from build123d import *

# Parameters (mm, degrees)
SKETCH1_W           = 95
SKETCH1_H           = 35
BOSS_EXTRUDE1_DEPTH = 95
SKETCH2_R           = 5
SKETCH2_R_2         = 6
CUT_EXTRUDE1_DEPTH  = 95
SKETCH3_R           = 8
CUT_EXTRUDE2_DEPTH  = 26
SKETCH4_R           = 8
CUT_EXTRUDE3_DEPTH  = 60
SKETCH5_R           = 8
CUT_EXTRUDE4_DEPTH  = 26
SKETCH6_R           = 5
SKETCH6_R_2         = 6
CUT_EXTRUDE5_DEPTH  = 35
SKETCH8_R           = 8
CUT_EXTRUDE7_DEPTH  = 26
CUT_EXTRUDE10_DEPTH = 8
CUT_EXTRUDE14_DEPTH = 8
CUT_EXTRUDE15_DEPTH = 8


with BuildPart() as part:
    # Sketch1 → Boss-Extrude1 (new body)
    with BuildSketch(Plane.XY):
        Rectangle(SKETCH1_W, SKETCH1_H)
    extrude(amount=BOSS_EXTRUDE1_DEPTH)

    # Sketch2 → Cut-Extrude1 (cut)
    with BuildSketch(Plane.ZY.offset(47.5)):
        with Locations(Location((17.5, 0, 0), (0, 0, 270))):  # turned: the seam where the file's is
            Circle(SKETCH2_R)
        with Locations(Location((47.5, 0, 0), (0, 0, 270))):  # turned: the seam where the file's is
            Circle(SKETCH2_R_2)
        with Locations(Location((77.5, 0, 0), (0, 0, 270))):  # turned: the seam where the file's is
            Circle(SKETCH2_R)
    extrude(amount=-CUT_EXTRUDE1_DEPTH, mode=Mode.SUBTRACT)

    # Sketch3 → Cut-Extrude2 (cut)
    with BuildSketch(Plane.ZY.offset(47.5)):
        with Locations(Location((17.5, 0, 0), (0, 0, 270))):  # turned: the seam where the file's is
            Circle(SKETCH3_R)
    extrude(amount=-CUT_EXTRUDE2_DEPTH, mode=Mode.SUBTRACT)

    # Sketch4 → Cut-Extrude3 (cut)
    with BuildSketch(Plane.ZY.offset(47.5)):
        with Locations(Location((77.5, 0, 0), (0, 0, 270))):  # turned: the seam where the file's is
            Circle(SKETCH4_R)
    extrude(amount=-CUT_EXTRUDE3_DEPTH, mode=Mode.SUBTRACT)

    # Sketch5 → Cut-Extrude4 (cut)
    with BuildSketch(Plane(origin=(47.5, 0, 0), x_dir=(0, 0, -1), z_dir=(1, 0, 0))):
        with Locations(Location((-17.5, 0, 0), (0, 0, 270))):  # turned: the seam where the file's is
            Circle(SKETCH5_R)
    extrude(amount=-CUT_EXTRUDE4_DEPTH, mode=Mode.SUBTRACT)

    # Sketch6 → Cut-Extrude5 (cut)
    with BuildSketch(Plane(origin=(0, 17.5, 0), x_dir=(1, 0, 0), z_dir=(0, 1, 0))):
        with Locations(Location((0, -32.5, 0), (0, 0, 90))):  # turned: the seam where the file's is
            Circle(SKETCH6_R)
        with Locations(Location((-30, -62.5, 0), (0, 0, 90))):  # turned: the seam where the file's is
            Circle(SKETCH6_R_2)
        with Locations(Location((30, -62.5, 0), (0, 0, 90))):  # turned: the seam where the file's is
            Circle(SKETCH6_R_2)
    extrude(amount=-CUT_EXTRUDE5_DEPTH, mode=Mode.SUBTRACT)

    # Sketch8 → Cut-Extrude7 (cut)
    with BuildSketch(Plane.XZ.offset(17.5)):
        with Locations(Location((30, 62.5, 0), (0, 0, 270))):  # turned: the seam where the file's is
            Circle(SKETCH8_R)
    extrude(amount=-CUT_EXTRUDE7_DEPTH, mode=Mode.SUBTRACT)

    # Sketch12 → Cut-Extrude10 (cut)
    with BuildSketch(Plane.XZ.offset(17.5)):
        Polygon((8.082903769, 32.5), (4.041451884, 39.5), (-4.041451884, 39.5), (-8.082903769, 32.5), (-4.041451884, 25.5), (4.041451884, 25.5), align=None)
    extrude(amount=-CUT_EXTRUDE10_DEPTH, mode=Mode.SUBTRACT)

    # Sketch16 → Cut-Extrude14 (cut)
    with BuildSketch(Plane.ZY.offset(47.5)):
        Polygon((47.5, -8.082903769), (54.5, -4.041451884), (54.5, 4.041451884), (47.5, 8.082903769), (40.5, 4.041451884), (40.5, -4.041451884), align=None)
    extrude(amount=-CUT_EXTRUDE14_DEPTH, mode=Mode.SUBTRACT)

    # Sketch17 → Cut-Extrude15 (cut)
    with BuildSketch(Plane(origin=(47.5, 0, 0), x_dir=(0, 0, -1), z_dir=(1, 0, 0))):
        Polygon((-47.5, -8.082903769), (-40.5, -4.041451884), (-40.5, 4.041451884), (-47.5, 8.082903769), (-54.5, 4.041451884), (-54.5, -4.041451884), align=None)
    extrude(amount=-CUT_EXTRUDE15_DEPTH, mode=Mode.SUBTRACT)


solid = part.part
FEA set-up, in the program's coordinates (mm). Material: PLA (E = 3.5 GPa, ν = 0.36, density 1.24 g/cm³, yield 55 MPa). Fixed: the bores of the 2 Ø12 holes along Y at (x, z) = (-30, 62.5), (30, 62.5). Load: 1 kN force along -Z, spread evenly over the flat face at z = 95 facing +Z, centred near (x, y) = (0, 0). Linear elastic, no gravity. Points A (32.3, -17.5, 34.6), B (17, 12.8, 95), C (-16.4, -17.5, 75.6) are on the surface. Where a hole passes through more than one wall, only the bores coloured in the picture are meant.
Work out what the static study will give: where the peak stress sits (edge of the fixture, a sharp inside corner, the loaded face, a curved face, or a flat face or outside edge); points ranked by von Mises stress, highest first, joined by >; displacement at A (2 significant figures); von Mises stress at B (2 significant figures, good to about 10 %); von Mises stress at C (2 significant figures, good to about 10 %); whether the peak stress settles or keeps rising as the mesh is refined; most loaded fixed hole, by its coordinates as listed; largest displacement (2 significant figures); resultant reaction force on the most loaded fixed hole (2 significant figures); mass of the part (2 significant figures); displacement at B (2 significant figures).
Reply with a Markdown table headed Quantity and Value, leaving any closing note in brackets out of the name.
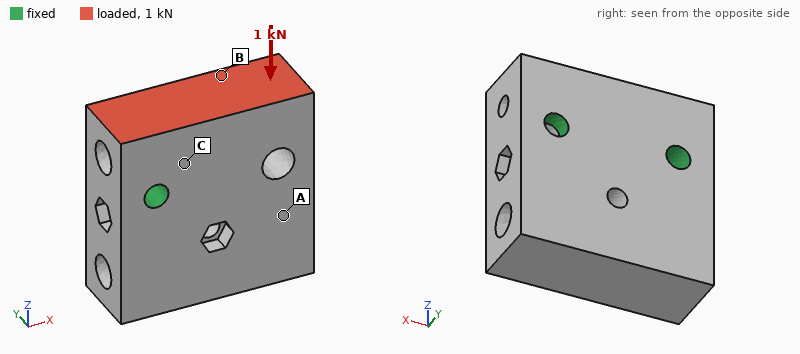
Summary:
| Quantity | Value |
|---|---|
| where the peak stress sits | edge of the fixture |
| points ranked by von Mises stress, highest first, joined by > | C > B > A |
| displacement at A | 15 µm |
| von Mises stress at B | 0.34 MPa |
| von Mises stress at C | 0.67 MPa |
| whether the peak stress settles or keeps rising as the mesh is refined | keeps rising |
| most loaded fixed hole, by its coordinates as listed | (-30, 62.5) |
| largest displacement | 24 µm |
| resultant reaction force on the most loaded fixed hole | 540 N |
| mass of the part | 320 g |
| displacement at B | 12 µm |
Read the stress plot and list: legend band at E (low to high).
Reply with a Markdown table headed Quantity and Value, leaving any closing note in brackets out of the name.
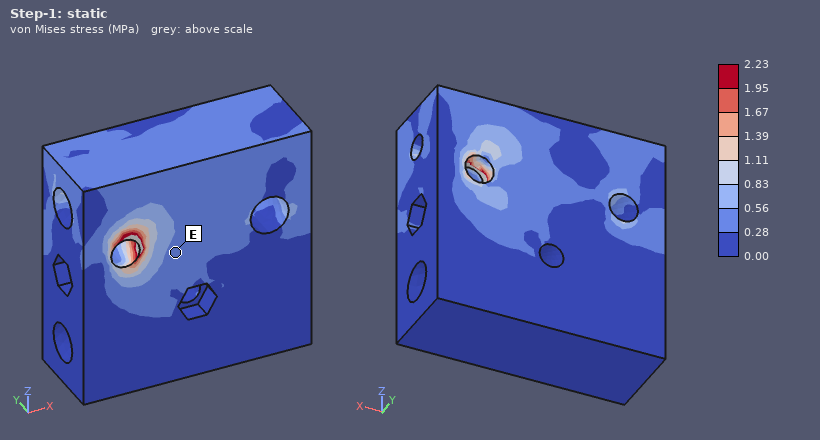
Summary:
| Quantity | Value |
|---|---|
| legend band at E | 0.28 to 0.56 MPa |
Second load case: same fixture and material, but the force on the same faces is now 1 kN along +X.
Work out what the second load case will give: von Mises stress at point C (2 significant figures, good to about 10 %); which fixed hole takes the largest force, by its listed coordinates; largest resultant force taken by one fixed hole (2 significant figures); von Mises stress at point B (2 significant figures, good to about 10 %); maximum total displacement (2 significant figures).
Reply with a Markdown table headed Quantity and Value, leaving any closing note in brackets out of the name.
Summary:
| Quantity | Value |
|---|---|
| von Mises stress at point C | 1.0 MPa |
| which fixed hole takes the largest force, by its listed coordinates | (-30, 62.5) |
| largest resultant force taken by one fixed hole | 820 N |
| von Mises stress at point B | 0.70 MPa |
| maximum total displacement | 35 µm |
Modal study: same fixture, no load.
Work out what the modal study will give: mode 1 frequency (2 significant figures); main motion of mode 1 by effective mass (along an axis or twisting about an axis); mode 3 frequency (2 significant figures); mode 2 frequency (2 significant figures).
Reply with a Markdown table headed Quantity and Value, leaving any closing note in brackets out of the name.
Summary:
| Quantity | Value |
|---|---|
| mode 1 frequency | 1300 Hz |
| main motion of mode 1 by effective mass | along Y |
| mode 3 frequency | 2600 Hz |
| mode 2 frequency | 2400 Hz |
